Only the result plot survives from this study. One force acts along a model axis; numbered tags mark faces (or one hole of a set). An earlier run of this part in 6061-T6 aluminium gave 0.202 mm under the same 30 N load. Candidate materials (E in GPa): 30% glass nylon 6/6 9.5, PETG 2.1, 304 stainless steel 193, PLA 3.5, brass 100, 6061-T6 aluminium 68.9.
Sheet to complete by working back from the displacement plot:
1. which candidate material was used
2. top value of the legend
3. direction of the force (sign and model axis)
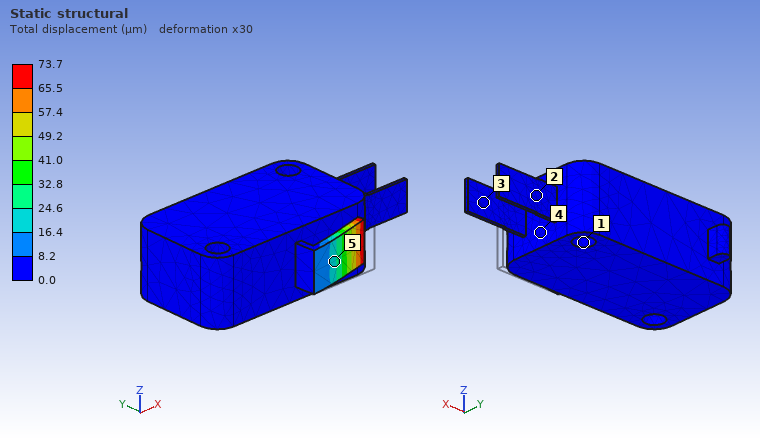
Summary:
304 stainless steel
73.7 µm
+Y
